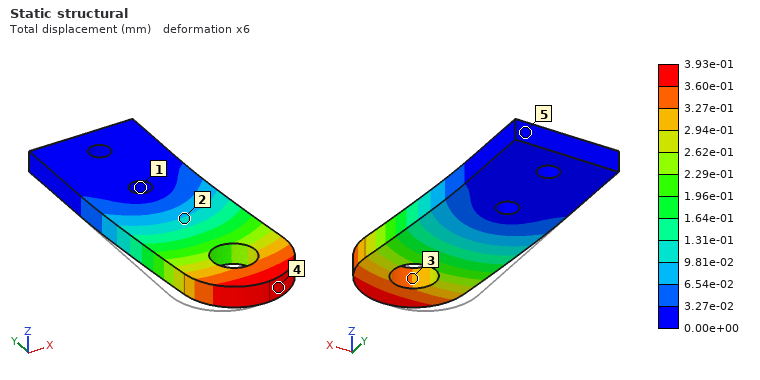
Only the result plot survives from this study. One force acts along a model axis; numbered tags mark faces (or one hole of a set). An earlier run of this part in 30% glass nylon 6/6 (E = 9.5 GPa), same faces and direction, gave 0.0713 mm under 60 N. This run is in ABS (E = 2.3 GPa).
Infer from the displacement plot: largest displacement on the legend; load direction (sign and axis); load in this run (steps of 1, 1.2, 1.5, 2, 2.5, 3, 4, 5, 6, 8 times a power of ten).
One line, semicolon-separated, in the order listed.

3.93e-01 mm; +X; 80 N
